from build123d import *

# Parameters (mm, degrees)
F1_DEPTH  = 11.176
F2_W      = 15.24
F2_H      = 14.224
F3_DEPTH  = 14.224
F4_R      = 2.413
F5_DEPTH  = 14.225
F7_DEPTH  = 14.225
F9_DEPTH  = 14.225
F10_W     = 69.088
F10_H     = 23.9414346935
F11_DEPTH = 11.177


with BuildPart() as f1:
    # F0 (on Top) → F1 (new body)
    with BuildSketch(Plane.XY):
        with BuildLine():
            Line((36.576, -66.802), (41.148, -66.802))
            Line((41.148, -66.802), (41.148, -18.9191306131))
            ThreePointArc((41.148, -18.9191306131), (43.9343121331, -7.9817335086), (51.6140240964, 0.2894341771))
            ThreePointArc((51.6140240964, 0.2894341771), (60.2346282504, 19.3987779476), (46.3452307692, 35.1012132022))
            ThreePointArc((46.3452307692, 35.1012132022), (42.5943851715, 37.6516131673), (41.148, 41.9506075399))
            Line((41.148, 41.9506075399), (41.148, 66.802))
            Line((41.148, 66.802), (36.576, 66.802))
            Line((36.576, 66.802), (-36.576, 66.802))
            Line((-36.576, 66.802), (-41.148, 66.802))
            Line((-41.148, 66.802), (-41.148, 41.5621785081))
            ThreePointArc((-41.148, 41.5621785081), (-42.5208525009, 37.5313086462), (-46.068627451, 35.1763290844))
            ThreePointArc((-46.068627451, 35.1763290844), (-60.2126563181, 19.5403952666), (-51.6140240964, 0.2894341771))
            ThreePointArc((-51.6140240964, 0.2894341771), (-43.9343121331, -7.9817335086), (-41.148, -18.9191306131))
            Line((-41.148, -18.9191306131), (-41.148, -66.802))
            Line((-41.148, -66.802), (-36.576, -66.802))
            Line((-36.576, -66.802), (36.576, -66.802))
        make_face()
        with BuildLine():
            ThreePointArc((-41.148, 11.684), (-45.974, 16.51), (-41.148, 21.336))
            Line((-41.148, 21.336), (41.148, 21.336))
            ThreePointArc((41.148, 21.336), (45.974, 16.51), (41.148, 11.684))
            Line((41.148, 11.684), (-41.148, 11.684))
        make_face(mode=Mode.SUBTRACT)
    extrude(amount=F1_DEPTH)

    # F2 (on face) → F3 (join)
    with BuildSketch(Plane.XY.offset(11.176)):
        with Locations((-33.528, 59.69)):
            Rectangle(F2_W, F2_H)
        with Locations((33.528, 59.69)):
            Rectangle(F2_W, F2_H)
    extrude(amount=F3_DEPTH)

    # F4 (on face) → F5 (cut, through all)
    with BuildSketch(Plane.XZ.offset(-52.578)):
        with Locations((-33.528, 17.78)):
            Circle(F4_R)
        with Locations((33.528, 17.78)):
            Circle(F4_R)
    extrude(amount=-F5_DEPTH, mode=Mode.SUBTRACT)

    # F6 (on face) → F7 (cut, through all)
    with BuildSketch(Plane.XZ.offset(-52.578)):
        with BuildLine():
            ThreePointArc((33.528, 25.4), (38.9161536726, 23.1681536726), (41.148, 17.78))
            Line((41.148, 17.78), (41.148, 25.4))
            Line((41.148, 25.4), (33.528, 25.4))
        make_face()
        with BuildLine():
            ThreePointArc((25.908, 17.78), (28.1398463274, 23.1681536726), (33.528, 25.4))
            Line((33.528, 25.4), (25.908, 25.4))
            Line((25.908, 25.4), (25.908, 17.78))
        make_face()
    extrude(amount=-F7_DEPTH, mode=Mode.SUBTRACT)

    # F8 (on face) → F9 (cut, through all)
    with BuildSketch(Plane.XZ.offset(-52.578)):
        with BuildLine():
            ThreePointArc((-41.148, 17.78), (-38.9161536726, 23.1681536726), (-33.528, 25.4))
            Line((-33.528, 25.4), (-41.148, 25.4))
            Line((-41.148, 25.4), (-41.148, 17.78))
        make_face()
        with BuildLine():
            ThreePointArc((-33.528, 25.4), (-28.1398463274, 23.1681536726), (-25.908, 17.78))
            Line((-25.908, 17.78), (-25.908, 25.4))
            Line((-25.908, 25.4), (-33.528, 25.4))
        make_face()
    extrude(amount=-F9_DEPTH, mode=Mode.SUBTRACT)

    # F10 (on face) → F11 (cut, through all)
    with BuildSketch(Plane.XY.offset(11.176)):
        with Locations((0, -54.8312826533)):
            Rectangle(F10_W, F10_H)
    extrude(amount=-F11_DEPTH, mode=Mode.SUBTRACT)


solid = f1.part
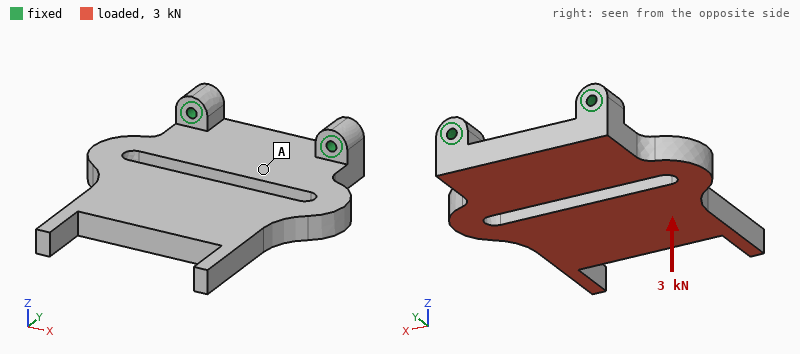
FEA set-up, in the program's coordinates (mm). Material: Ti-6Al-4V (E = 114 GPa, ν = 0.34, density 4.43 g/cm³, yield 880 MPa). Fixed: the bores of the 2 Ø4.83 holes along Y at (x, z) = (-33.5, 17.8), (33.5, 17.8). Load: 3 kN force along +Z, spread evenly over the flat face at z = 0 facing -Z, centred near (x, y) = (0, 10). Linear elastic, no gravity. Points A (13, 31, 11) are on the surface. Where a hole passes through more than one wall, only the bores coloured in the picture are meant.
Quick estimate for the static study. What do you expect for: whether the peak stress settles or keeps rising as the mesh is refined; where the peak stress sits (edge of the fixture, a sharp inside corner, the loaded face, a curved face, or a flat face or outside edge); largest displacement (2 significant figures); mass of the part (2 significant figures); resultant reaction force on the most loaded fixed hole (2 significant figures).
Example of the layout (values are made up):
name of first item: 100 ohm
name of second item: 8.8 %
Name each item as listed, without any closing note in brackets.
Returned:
whether the peak stress settles or keeps rising as the mesh is refined: keeps rising
where the peak stress sits: edge of the fixture
largest displacement: 1.3 mm
mass of the part: 500 g
resultant reaction force on the most loaded fixed hole: 1.6 kN
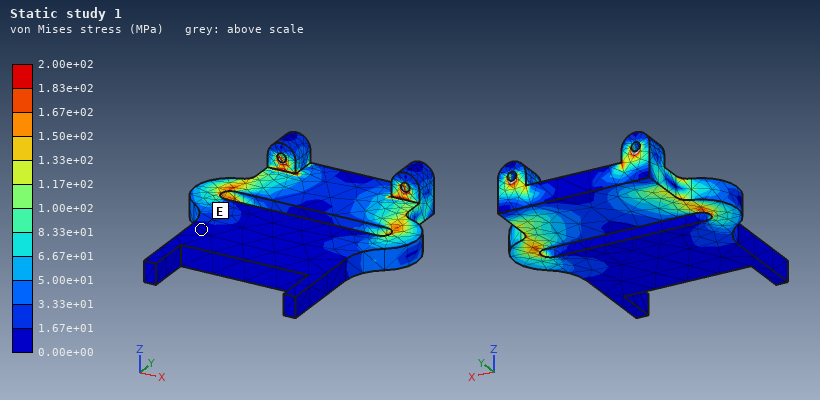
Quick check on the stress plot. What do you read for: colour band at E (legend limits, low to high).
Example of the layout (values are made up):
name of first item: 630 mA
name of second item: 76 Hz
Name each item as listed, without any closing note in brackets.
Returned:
colour band at E: 0.00e+00 to 1.67e+01 MPa
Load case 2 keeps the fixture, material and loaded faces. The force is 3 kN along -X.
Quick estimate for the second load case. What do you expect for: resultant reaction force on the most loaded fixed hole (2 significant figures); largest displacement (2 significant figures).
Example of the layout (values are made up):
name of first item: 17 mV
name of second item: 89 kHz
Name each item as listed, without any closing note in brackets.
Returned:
resultant reaction force on the most loaded fixed hole: 2.6 kN
largest displacement: 63 µm
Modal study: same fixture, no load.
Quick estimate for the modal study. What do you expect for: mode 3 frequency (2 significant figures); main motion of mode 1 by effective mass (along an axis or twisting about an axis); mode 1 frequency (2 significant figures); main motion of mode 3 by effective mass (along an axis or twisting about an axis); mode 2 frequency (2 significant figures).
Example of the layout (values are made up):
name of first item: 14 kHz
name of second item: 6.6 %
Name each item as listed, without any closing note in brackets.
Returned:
mode 3 frequency: 2000 Hz
main motion of mode 1 by effective mass: along Z
mode 1 frequency: 470 Hz
main motion of mode 3 by effective mass: along X
mode 2 frequency: 1700 Hz
